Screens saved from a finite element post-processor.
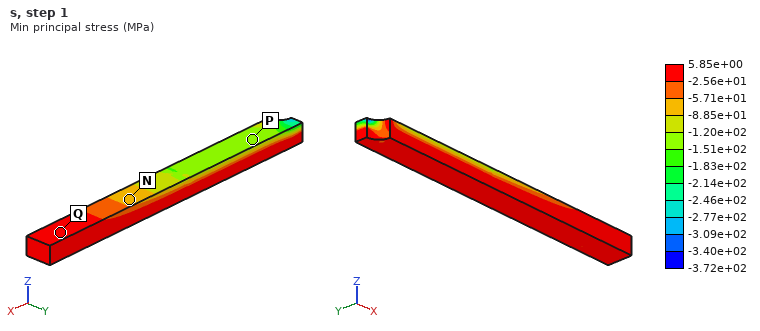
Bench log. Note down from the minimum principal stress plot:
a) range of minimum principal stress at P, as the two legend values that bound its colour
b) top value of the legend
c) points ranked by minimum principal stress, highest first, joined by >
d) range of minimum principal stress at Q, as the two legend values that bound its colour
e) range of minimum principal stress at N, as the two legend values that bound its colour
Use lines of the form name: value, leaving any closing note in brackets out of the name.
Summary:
range of minimum principal stress at P, as the two legend values that bound its colour: -1.51e+02 to -1.20e+02 MPa
top value of the legend: 5.85e+00 MPa
points ranked by minimum principal stress, highest first, joined by >: Q > N > P
range of minimum principal stress at Q, as the two legend values that bound its colour: -2.56e+01 to 5.85e+00 MPa
range of minimum principal stress at N, as the two legend values that bound its colour: -8.85e+01 to -5.71e+01 MPa
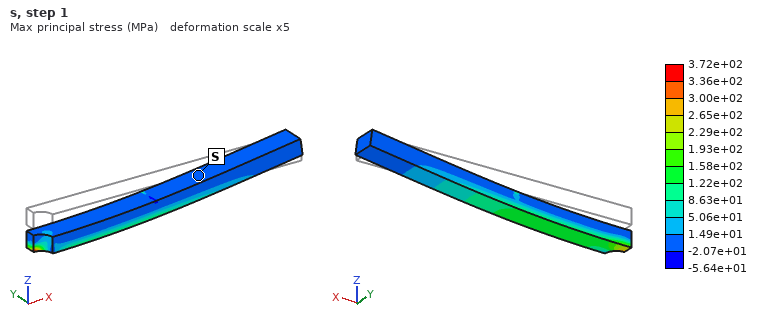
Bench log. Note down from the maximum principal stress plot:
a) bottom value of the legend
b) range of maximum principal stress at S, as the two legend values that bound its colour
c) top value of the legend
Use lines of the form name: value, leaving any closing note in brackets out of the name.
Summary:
bottom value of the legend: -5.64e+01 MPa
range of maximum principal stress at S, as the two legend values that bound its colour: -2.07e+01 to 1.49e+01 MPa
top value of the legend: 3.72e+02 MPa
